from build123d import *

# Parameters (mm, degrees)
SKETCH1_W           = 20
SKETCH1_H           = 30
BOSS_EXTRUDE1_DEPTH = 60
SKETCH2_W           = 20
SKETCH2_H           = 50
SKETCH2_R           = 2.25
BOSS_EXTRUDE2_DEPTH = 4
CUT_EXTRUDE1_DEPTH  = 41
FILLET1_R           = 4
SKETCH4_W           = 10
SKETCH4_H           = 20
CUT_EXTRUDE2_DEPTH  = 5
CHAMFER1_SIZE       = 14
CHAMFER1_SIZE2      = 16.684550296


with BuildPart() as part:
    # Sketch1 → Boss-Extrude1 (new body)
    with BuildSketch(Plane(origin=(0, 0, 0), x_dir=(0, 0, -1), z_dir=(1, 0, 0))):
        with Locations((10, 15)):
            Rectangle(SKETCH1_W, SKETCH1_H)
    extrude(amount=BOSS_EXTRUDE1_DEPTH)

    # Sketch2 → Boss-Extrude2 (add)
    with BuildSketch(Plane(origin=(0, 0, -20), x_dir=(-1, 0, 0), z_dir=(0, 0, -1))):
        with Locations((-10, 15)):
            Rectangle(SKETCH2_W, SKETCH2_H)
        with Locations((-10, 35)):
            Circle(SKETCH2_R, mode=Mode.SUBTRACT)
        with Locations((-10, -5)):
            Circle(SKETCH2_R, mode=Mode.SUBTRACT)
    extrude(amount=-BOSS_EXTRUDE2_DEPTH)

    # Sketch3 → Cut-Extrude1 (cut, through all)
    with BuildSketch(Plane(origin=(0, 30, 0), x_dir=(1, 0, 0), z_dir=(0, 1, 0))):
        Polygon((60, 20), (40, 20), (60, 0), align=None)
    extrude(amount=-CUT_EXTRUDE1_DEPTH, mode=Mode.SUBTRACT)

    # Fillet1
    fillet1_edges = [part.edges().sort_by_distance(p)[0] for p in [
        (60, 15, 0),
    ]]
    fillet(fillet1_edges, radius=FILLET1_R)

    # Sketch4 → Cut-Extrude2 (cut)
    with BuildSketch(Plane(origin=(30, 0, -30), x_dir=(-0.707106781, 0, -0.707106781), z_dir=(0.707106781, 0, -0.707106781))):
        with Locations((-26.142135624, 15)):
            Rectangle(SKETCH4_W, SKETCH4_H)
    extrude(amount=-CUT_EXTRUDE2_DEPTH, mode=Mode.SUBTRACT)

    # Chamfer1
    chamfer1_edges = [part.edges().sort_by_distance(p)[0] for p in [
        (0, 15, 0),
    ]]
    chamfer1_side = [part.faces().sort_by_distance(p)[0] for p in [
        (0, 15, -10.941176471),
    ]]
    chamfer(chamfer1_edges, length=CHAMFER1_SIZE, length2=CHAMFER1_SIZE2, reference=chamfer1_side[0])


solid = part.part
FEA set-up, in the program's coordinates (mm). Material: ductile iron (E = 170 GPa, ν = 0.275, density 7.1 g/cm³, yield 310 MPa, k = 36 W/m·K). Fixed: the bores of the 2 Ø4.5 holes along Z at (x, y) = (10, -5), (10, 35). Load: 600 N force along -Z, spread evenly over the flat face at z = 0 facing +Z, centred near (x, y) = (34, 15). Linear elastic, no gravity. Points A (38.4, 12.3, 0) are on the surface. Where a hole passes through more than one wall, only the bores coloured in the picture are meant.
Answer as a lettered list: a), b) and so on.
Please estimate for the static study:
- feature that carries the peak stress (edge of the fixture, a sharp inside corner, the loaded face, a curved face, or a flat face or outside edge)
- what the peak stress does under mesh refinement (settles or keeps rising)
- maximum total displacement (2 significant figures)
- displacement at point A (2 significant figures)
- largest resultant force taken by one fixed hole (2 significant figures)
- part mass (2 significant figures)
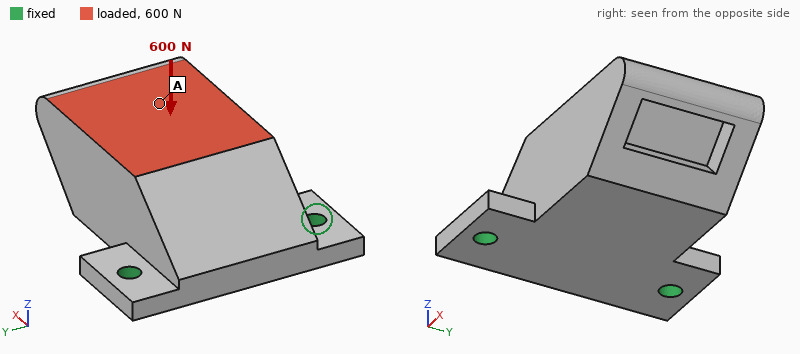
a) edge of the fixture
b) keeps rising
c) 65 µm
d) 47 µm
e) 330 N
f) 190 g
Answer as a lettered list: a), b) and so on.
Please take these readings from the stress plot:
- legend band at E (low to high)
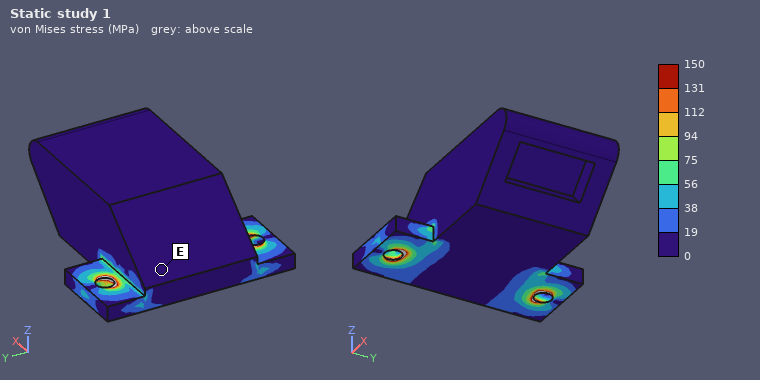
a) 0 to 19 MPa
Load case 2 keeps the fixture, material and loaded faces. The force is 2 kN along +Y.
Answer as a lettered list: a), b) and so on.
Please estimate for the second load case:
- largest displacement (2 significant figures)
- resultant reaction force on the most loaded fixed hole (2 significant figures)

a) 15 µm
b) 1.9 kN
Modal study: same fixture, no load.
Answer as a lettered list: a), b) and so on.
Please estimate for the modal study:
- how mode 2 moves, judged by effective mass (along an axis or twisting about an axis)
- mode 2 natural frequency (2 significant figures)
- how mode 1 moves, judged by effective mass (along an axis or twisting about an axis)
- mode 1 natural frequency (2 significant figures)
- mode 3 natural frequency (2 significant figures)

a) along Y
b) 7500 Hz
c) along Z
d) 1600 Hz
e) 10 kHz
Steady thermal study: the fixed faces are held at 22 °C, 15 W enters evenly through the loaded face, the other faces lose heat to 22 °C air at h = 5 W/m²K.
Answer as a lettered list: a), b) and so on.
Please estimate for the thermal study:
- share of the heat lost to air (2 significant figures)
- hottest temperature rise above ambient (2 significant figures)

a) 5.2 %
b) 42 K
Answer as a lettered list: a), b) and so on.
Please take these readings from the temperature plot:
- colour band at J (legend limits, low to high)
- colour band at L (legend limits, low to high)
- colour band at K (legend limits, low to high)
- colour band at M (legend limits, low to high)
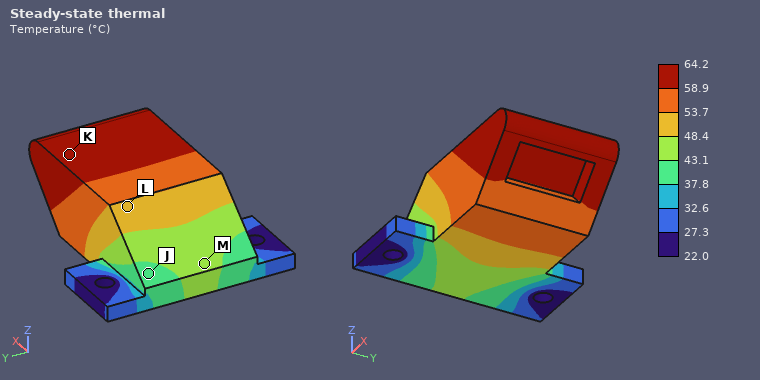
a) 37.8 to 43.1 °C
b) 48.4 to 53.7 °C
c) 58.9 to 64.2 °C
d) 43.1 to 48.4 °C
